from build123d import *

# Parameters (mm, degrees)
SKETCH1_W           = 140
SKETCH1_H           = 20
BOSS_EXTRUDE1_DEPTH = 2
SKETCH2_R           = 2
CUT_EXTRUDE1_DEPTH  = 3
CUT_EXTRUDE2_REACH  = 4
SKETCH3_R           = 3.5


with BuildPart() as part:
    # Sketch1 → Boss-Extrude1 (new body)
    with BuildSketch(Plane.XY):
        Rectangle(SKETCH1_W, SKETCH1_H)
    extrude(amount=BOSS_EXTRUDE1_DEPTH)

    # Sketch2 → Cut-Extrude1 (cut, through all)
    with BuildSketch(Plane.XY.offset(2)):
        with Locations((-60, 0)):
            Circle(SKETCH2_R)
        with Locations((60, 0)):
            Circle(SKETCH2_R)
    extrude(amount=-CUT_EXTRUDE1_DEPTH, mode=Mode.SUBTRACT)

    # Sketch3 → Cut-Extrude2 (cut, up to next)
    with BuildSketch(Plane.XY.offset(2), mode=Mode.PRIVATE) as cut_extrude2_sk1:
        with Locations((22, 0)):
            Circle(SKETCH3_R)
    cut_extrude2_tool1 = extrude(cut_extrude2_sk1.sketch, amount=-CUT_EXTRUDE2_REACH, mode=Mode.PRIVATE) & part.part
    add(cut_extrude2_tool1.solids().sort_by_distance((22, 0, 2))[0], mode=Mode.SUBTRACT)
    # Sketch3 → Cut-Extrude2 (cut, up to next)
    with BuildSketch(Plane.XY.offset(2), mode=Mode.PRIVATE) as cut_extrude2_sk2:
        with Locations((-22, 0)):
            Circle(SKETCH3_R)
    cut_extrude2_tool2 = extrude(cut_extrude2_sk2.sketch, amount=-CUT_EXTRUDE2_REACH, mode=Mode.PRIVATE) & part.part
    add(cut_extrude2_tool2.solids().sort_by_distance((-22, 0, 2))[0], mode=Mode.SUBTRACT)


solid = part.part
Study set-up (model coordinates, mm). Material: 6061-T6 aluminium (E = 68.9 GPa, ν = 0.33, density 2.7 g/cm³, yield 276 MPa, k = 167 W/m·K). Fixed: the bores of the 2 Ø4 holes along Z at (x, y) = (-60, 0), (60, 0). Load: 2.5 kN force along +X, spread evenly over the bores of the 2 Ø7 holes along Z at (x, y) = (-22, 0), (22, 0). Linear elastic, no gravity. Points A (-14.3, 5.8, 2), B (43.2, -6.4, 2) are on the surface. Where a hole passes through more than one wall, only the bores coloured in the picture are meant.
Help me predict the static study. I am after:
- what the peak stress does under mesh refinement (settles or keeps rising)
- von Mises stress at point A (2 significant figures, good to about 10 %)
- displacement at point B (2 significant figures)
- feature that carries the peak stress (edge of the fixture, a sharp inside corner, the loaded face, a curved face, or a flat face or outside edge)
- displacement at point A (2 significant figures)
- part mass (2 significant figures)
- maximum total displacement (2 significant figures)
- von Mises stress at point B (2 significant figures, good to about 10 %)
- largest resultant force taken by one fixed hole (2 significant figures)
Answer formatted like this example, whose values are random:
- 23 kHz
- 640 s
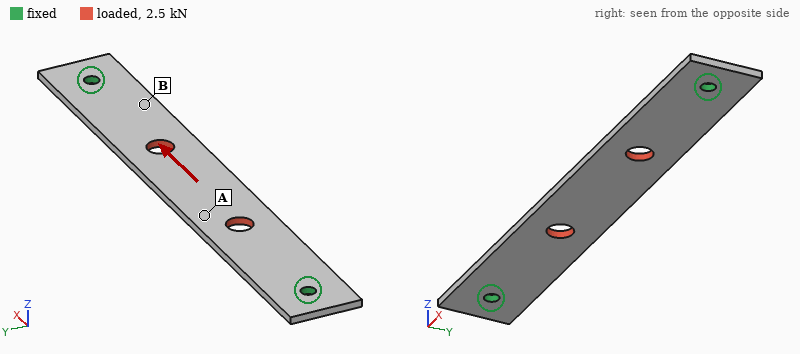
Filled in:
- keeps rising
- 11 MPa
- 9.8 µm
- edge of the fixture
- 21 µm
- 15 g
- 23 µm
- 31 MPa
- 1.3 kN
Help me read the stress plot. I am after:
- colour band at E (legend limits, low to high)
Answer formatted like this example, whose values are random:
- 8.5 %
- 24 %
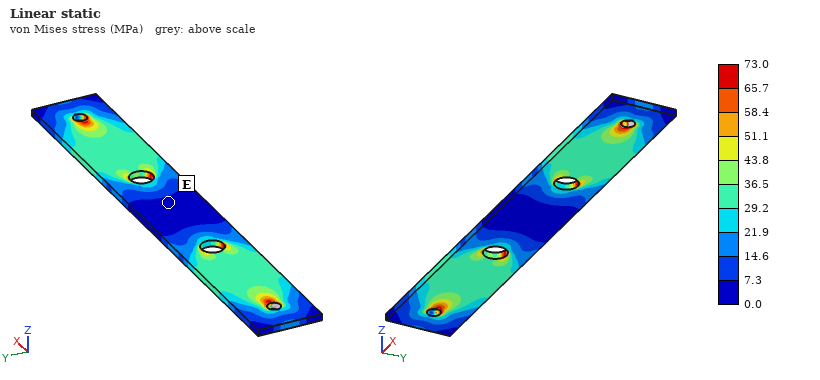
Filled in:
- 0.0 to 7.3 MPa
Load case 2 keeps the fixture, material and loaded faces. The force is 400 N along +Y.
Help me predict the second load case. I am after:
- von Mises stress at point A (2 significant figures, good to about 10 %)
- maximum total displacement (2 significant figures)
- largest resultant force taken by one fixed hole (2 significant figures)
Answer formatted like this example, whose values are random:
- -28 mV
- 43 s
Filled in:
- 17 MPa
- 72 µm
- 200 N
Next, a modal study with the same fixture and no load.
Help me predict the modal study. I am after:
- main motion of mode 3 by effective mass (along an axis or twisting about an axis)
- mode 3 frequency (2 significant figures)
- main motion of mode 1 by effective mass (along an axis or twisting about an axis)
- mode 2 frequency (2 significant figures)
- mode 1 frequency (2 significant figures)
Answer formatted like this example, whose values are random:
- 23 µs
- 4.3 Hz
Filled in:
- twisting about X
- 2500 Hz
- along Z
- 2000 Hz
- 750 Hz
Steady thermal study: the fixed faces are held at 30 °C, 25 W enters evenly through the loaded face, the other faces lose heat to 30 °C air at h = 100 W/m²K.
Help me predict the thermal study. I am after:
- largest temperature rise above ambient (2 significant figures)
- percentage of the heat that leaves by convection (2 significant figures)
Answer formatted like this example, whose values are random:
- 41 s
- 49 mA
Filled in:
- 44 K
- 53 %
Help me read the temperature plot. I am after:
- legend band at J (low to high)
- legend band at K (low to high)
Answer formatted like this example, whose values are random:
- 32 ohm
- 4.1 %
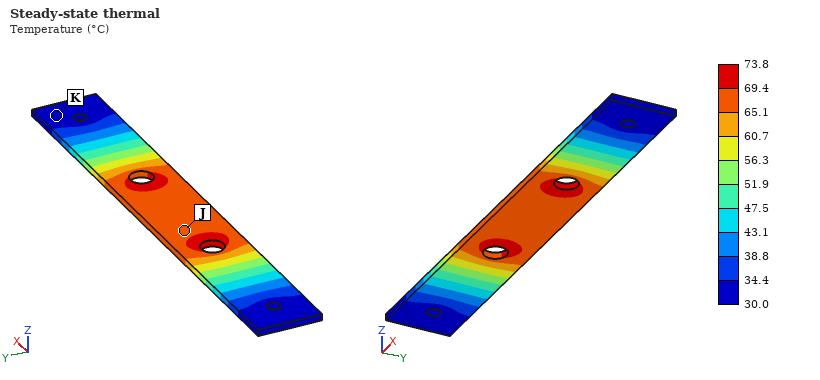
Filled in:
- 65.1 to 69.4 °C
- 30.0 to 34.4 °C
